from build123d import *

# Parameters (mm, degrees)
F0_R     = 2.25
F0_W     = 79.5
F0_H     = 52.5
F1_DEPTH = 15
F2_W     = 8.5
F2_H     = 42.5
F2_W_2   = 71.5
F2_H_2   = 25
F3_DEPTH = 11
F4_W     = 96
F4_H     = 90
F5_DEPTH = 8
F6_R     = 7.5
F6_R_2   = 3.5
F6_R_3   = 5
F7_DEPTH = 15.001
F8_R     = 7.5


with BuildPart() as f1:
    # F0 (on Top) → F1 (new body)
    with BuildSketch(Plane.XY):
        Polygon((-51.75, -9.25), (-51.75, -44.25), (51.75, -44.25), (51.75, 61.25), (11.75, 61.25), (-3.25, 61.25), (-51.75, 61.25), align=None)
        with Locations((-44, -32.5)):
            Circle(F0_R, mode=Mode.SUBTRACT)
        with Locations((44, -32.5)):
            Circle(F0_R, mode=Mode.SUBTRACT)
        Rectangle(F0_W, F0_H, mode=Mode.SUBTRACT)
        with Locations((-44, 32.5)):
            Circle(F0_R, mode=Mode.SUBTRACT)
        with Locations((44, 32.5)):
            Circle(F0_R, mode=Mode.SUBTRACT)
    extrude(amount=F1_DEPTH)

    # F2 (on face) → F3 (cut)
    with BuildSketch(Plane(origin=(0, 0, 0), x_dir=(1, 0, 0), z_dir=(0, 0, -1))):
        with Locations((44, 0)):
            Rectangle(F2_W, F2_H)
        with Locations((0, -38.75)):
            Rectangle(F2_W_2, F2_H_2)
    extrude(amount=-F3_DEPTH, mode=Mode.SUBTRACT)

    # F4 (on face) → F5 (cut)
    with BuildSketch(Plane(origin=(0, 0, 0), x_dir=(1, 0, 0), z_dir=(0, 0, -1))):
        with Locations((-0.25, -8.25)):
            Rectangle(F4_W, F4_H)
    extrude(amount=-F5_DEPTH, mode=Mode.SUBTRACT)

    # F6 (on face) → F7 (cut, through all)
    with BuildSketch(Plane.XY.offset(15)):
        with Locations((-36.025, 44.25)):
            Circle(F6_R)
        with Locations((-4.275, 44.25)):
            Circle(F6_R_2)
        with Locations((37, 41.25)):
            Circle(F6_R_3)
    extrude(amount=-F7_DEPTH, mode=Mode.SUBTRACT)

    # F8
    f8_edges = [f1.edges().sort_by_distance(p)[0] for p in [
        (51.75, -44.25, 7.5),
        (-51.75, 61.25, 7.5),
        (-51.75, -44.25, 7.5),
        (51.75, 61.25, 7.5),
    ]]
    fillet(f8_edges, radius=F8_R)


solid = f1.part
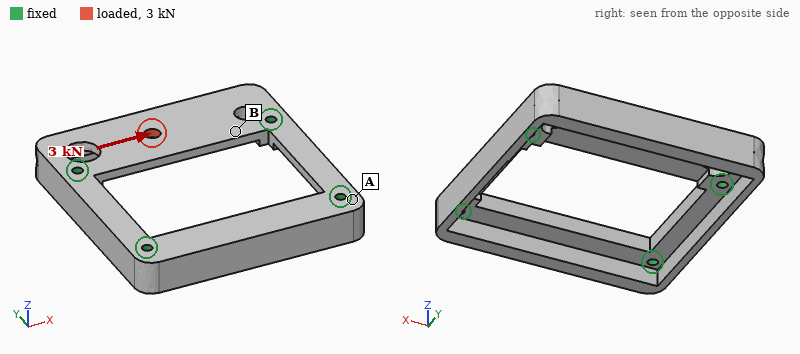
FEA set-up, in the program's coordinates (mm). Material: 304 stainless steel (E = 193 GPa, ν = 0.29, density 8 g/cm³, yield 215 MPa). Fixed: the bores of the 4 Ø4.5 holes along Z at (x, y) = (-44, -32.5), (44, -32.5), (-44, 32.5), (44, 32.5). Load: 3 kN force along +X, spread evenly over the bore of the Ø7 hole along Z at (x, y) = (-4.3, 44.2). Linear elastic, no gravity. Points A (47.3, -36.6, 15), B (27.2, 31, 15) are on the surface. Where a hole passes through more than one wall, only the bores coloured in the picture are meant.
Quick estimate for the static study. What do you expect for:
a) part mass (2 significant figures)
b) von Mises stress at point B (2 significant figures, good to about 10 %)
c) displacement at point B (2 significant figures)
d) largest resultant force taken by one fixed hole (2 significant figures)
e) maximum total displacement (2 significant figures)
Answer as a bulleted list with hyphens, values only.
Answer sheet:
- 450 g
- 19 MPa
- 2.0 µm
- 1.5 kN
- 5.7 µm
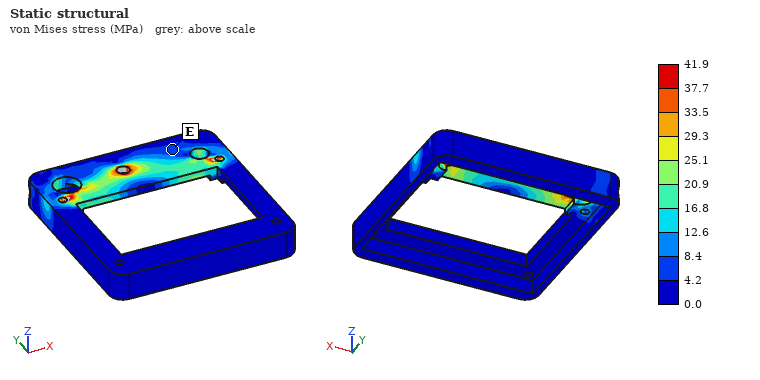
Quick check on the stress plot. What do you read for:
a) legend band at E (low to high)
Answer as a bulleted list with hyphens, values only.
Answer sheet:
- 4.2 to 8.4 MPa
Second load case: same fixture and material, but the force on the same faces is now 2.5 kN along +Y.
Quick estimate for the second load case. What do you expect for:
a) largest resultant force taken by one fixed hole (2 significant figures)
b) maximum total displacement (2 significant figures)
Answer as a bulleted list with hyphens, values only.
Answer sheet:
- 1.7 kN
- 15 µm
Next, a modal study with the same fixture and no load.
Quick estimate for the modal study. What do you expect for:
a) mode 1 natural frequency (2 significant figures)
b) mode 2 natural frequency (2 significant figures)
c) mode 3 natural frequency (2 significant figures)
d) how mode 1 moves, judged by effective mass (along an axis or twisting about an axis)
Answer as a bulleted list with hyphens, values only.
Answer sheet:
- 2800 Hz
- 4800 Hz
- 5200 Hz
- along Z
